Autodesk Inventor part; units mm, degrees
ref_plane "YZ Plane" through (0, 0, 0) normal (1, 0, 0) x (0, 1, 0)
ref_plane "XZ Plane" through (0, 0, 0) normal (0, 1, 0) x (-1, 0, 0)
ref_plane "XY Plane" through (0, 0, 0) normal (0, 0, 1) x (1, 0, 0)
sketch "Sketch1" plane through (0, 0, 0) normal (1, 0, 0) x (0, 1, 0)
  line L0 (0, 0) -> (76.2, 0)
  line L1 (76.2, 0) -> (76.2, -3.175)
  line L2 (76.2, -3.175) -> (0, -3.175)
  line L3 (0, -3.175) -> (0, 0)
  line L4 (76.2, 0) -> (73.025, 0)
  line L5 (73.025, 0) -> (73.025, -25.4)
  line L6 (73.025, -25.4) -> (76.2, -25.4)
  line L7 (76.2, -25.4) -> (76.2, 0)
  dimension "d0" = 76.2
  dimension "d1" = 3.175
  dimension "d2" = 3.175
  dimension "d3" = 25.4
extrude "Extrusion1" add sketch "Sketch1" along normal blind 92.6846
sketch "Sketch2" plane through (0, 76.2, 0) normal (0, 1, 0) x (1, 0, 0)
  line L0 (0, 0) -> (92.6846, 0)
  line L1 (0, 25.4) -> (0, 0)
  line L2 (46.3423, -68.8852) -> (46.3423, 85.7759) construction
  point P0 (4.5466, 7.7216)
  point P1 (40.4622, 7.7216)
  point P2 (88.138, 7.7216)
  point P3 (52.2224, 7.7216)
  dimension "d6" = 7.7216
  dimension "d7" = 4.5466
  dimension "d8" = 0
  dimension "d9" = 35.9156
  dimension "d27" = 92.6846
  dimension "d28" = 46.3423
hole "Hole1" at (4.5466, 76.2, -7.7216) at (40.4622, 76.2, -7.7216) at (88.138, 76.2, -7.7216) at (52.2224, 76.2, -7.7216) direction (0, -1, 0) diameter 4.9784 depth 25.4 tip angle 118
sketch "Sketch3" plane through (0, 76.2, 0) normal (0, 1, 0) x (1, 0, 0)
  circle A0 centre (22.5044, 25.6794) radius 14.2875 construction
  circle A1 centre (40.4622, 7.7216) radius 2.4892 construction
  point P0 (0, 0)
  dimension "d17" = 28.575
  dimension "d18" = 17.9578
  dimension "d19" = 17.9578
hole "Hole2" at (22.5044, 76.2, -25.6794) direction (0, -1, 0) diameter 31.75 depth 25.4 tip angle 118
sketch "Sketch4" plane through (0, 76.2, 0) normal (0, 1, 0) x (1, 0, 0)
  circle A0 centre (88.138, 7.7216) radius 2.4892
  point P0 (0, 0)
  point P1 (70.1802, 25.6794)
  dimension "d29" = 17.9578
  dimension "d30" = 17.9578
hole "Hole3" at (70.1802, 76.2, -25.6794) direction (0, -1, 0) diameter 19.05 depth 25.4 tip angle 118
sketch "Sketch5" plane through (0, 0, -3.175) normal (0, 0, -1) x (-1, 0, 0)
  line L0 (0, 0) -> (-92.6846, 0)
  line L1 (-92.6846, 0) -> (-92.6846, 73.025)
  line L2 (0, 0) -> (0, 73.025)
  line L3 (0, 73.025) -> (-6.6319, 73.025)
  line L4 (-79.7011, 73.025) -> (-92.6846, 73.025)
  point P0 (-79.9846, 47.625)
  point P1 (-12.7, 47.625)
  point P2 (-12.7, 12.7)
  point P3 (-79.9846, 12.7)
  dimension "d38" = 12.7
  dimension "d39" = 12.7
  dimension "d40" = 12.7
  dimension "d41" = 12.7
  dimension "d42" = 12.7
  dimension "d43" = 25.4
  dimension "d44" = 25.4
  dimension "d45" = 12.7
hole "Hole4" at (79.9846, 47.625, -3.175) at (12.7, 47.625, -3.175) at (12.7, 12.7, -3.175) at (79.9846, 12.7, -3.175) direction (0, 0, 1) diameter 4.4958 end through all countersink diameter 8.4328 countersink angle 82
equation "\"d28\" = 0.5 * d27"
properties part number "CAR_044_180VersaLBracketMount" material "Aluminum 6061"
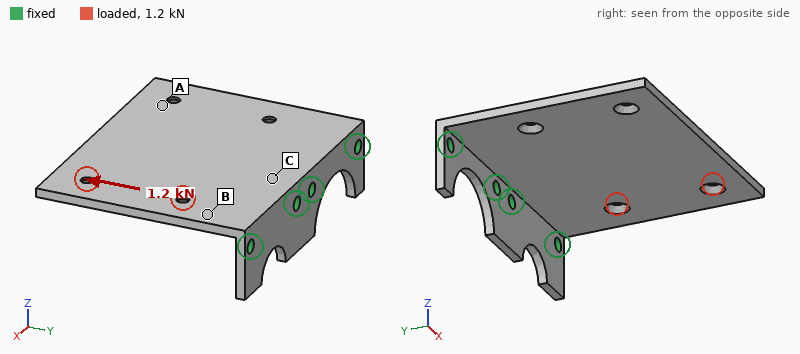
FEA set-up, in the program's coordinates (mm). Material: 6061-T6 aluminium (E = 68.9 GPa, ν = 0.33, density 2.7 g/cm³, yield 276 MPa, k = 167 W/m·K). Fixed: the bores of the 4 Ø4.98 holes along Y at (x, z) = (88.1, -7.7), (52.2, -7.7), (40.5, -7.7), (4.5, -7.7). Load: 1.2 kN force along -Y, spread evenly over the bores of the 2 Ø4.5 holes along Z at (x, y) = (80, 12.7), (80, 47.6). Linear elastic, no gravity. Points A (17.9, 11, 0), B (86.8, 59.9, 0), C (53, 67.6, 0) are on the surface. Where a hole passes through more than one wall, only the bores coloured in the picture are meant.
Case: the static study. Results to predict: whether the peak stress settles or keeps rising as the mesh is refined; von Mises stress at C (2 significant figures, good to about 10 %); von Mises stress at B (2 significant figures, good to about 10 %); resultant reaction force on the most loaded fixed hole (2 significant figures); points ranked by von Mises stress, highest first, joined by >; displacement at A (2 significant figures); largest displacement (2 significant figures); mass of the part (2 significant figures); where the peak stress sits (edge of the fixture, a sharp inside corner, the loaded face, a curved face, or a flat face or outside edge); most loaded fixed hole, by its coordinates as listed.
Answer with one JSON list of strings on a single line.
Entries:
["keeps rising", "18 MPa", "24 MPa", "800 N", "B > C > A", "0.16 mm", "0.40 mm", "72 g", "edge of the fixture", "(88.1, -7.7)"]
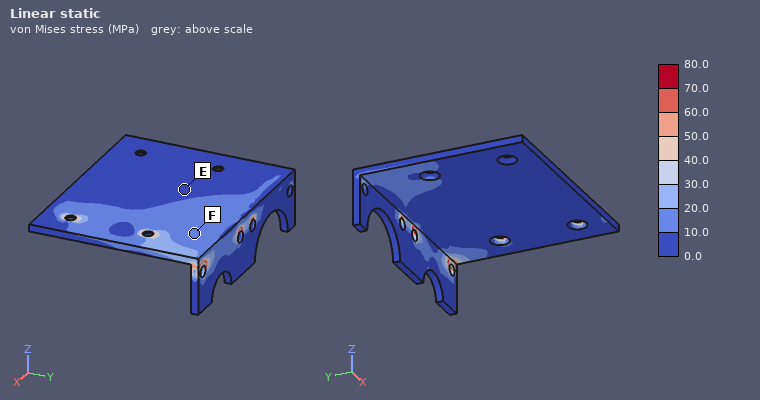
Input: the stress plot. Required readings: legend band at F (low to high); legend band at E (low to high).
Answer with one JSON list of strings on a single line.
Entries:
["10.0 to 20.0 MPa", "0.0 to 10.0 MPa"]
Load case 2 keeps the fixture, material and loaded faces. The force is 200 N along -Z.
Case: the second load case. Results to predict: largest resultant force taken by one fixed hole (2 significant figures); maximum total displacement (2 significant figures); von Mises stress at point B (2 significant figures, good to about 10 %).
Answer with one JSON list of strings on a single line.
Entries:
["110 N", "1.3 mm", "52 MPa"]
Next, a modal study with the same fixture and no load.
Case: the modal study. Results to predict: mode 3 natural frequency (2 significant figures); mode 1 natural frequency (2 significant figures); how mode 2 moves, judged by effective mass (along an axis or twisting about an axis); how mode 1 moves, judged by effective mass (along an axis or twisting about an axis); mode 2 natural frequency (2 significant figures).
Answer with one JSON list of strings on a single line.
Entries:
["2400 Hz", "430 Hz", "twisting about Y", "along Z", "930 Hz"]
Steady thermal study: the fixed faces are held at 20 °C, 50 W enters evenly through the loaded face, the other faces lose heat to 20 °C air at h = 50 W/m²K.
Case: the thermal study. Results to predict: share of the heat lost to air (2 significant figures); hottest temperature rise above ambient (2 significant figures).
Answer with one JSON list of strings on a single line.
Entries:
["37 %", "74 K"]
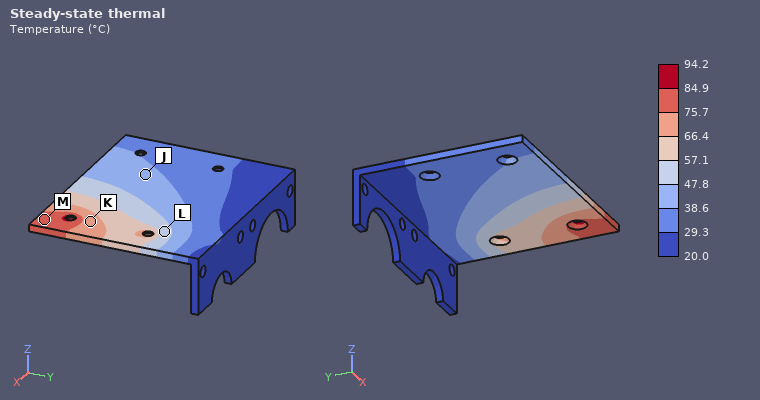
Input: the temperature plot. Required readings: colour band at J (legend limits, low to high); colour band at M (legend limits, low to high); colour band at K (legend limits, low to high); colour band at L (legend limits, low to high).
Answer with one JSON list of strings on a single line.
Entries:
["38.6 to 47.8 °C", "75.7 to 84.9 °C", "66.4 to 75.7 °C", "47.8 to 57.1 °C"]
